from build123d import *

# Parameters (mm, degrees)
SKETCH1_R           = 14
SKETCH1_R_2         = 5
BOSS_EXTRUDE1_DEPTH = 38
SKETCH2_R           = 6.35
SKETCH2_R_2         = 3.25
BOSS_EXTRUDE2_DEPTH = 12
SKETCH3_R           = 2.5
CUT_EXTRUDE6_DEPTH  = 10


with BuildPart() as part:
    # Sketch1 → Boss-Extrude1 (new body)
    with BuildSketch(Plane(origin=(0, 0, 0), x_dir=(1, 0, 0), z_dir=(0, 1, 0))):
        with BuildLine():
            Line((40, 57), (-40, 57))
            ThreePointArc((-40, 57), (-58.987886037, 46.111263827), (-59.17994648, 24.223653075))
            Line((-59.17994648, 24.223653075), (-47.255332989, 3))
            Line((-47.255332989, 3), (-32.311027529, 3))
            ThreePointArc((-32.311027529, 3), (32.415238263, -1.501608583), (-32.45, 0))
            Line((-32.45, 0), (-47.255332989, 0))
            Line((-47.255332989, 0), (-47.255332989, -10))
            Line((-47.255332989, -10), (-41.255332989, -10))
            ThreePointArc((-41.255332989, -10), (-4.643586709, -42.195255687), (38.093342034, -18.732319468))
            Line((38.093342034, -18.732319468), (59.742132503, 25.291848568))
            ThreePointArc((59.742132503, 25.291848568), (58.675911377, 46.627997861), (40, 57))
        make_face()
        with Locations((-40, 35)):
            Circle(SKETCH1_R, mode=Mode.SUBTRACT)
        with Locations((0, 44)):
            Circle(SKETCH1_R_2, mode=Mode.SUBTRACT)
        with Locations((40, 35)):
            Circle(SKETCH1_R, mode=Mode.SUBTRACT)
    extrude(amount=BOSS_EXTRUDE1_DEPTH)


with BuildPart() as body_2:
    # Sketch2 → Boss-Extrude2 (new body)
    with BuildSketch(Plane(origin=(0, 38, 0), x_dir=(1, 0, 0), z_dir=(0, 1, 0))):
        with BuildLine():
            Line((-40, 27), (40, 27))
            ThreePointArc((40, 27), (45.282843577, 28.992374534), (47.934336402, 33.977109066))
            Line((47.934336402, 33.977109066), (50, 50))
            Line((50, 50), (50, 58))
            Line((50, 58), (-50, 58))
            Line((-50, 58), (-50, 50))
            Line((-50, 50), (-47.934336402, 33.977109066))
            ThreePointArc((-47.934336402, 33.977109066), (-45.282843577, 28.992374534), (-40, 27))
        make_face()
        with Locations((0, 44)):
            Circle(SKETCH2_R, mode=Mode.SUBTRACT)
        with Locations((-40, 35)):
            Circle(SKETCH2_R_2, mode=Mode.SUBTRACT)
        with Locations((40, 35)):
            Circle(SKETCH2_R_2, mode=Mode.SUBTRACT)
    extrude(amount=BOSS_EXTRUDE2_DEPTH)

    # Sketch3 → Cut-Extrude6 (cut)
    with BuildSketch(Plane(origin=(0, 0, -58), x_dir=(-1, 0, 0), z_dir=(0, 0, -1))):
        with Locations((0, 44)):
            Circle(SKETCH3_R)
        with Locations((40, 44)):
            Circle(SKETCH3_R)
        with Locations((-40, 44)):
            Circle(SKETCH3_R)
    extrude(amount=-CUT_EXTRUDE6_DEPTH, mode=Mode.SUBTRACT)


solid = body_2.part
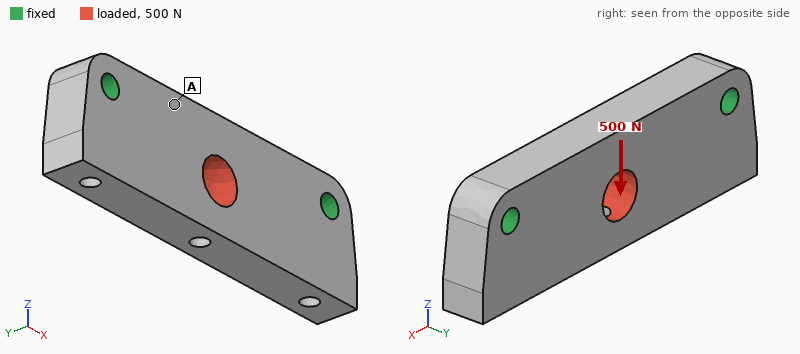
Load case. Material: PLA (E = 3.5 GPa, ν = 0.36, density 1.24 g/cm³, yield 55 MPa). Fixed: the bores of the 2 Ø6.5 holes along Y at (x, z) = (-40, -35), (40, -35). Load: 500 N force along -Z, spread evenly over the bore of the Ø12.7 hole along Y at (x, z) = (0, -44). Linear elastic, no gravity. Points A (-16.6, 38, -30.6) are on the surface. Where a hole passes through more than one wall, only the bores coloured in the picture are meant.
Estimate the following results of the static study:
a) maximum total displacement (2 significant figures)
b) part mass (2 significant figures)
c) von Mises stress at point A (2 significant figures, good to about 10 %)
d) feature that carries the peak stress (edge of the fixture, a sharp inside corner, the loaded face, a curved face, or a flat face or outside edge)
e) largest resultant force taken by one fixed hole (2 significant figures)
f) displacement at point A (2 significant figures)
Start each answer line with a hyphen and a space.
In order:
- 56 µm
- 41 g
- 0.96 MPa
- a curved face
- 290 N
- 37 µm
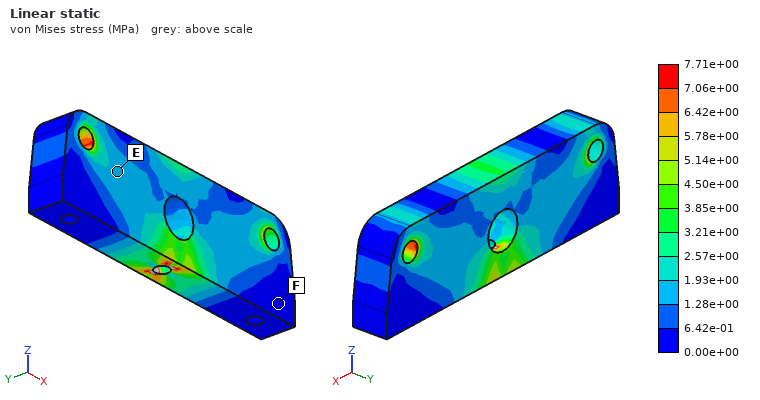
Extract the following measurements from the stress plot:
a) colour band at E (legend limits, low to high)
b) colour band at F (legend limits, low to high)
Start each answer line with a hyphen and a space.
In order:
- 1.28e+00 to 1.93e+00 MPa
- 0.00e+00 to 6.42e-01 MPa
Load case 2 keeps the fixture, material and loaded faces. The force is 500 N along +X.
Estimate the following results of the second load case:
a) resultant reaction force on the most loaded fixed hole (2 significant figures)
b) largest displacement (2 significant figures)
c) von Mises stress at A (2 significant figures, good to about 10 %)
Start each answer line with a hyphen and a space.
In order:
- 250 N
- 13 µm
- 0.77 MPa
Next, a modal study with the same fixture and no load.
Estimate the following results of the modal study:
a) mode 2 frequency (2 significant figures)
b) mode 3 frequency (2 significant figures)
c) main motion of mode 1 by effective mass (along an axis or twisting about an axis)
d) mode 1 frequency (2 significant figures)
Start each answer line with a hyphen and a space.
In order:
- 3800 Hz
- 3800 Hz
- along Y
- 2400 Hz
